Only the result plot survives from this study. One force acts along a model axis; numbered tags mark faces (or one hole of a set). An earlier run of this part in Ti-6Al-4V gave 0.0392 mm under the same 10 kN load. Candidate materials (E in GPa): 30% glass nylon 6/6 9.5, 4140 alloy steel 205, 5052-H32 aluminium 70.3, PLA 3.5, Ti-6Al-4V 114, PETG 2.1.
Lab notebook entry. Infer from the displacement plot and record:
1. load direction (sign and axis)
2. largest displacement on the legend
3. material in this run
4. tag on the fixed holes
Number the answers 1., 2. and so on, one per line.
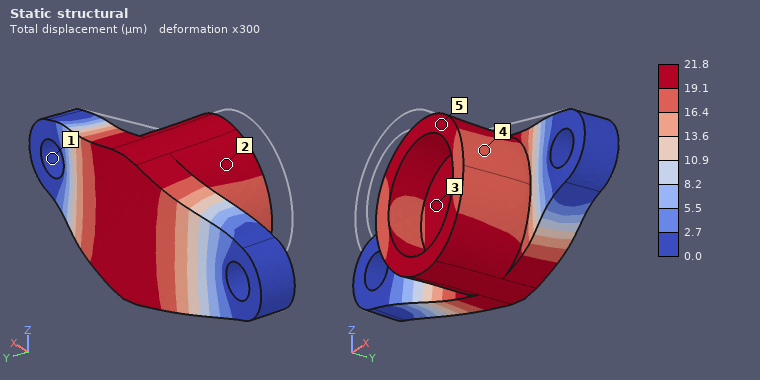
1. +Y
2. 21.8 µm
3. 4140 alloy steel
4. 1
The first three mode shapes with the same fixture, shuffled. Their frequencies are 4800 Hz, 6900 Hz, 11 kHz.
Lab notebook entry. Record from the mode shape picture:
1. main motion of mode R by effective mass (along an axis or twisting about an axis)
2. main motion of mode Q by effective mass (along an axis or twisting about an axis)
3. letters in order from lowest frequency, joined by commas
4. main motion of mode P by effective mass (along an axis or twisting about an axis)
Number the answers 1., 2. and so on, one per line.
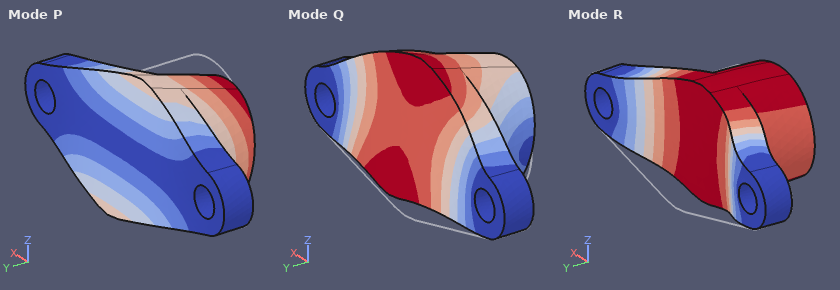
1. along Y
2. along Z
3. P, R, Q
4. along Z
